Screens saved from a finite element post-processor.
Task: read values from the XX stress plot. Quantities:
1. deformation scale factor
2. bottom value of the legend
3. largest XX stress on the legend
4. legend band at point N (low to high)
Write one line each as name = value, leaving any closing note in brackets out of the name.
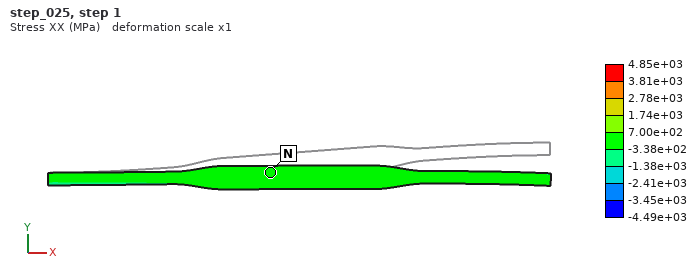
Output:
deformation scale factor = 1
bottom value of the legend = -4.49e+03 MPa
largest XX stress on the legend = 4.85e+03 MPa
legend band at point N = -3.38e+02 to 7.00e+02 MPa
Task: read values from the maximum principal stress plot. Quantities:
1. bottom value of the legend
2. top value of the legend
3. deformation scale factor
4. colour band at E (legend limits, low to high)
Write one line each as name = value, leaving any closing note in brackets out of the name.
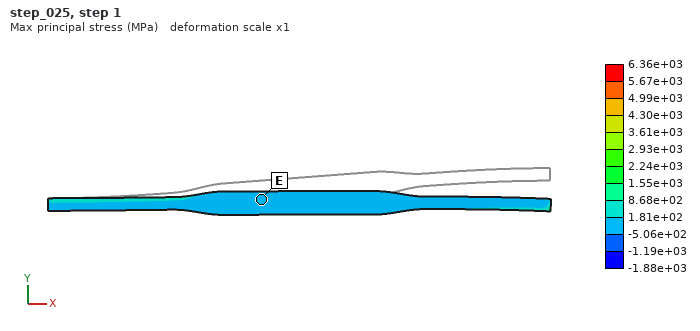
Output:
bottom value of the legend = -1.88e+03 MPa
top value of the legend = 6.36e+03 MPa
deformation scale factor = 1
colour band at E = -5.06e+02 to 1.81e+02 MPa
